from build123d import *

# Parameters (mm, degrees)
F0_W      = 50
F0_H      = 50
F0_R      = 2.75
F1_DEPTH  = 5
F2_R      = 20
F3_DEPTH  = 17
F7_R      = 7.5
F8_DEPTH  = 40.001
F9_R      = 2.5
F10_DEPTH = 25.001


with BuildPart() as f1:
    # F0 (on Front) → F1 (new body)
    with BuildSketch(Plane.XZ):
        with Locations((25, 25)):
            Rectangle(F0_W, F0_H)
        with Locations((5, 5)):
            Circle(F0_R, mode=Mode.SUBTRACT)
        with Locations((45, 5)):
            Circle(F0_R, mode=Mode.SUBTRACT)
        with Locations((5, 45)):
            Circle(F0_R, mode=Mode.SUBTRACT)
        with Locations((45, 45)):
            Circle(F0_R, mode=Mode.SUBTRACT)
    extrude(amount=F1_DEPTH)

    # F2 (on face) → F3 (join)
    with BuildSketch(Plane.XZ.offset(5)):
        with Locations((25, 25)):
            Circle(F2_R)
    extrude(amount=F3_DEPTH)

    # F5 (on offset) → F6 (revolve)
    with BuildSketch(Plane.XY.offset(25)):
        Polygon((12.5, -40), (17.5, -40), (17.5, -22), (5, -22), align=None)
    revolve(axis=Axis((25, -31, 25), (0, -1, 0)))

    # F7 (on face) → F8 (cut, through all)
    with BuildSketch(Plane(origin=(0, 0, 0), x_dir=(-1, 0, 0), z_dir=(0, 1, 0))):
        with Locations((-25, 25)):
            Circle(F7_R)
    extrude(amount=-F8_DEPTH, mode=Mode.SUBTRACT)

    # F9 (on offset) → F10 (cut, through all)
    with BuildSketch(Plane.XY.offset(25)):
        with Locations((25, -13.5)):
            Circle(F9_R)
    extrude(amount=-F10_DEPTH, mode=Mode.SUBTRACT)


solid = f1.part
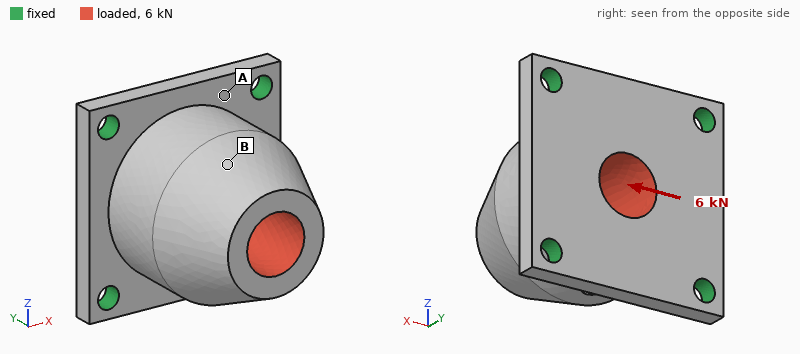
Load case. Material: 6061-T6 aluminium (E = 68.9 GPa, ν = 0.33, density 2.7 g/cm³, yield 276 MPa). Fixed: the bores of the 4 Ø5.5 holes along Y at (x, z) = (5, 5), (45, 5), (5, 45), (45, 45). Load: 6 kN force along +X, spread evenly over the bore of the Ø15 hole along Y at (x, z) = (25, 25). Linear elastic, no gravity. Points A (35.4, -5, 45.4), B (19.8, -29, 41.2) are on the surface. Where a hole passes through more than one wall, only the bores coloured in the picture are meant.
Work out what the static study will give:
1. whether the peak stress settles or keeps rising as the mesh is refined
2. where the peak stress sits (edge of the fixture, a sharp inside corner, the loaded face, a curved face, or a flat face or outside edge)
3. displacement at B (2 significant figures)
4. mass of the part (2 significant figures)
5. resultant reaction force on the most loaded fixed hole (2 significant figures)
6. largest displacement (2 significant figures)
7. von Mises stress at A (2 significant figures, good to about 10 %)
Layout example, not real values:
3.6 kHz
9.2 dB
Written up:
keeps rising
edge of the fixture
36 µm
110 g
2.3 kN
52 µm
40 MPa
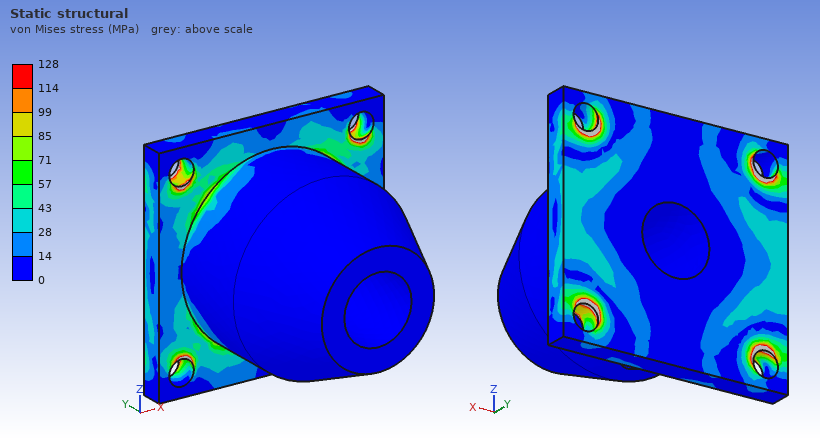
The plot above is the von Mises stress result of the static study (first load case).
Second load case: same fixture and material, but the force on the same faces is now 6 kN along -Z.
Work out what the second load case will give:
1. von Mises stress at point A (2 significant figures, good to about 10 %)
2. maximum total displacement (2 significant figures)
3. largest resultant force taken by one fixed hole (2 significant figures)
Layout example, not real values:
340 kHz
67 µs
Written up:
36 MPa
52 µm
2.3 kN
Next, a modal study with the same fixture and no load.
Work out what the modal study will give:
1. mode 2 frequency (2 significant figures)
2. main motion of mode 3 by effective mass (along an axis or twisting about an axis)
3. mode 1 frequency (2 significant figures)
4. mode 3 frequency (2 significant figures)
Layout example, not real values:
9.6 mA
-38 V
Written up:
7100 Hz
along Y
7100 Hz
9000 Hz
